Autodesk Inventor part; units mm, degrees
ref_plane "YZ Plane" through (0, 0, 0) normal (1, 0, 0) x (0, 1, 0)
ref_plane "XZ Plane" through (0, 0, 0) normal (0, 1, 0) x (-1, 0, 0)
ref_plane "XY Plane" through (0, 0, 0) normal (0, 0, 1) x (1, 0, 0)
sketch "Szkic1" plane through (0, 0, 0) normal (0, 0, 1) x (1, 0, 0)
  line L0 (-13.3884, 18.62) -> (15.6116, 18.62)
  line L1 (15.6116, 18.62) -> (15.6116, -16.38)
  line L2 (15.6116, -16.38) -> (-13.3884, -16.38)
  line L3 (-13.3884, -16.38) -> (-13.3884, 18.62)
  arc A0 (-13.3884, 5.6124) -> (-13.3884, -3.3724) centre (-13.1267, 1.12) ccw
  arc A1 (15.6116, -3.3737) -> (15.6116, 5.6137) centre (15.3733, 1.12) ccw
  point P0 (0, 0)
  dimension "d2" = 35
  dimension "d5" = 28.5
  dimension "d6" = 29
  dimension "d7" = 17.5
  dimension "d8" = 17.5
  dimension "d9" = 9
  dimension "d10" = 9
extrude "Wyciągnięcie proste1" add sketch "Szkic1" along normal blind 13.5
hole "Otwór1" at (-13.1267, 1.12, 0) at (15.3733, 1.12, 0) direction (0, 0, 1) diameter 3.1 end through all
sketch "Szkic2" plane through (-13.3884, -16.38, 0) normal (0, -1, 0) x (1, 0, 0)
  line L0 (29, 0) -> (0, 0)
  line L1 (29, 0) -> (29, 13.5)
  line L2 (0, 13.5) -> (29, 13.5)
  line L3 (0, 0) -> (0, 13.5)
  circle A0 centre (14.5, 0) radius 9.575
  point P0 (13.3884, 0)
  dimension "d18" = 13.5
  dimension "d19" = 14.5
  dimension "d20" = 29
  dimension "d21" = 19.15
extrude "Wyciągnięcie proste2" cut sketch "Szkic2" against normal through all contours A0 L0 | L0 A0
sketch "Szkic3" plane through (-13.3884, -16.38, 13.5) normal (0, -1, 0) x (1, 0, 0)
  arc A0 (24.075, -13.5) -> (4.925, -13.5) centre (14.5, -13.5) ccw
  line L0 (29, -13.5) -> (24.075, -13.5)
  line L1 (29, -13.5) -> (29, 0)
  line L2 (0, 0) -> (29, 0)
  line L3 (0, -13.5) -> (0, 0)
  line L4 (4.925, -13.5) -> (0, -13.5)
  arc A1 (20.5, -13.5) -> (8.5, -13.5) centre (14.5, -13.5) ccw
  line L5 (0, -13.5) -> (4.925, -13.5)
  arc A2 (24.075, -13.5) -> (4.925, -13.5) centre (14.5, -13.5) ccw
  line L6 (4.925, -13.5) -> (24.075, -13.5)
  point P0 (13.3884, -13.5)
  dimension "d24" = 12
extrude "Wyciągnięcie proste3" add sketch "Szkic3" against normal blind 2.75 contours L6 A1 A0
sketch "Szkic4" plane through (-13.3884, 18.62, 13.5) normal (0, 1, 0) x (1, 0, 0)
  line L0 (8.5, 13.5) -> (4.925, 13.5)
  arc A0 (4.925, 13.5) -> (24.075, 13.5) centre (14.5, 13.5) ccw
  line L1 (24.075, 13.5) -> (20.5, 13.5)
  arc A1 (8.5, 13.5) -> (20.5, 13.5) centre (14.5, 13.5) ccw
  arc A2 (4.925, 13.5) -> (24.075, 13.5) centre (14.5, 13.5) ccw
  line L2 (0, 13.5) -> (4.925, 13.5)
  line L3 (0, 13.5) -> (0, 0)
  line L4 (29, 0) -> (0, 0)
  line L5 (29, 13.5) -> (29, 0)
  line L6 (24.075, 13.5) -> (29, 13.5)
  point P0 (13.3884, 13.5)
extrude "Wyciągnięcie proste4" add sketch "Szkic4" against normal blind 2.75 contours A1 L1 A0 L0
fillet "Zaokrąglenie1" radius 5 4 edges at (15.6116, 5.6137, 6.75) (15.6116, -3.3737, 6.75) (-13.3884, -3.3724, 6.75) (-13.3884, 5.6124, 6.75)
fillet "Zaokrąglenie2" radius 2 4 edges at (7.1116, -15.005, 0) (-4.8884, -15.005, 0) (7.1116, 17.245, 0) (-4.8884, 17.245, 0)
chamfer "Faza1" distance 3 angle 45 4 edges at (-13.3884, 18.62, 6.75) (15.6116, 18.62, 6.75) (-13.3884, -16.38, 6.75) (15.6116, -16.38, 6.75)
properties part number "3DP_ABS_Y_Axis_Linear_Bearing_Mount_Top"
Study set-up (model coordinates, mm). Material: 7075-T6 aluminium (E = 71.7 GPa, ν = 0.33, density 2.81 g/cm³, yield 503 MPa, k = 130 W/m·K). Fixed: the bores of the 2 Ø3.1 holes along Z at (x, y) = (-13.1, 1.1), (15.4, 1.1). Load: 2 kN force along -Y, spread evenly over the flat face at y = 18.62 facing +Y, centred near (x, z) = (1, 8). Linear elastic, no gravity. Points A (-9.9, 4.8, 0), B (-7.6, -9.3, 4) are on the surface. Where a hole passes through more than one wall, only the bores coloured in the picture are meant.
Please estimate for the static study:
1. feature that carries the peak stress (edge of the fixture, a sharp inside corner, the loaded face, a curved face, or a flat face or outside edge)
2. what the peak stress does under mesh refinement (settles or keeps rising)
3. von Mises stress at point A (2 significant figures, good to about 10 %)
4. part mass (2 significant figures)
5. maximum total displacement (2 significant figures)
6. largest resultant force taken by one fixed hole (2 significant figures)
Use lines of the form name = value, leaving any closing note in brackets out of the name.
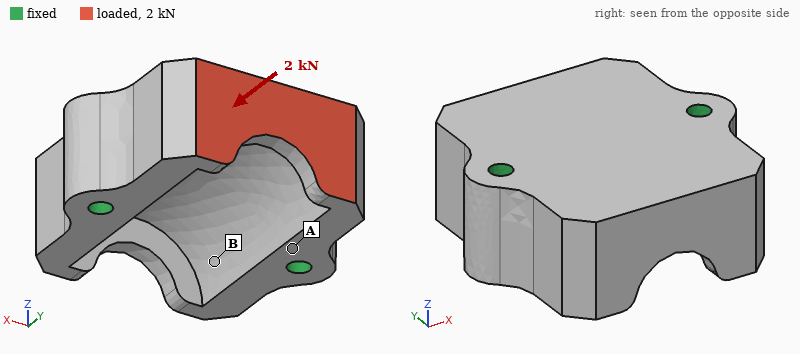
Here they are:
feature that carries the peak stress = a sharp inside corner
what the peak stress does under mesh refinement = keeps rising
von Mises stress at point A = 8.1 MPa
part mass = 27 g
maximum total displacement = 8.6 µm
largest resultant force taken by one fixed hole = 1.0 kN
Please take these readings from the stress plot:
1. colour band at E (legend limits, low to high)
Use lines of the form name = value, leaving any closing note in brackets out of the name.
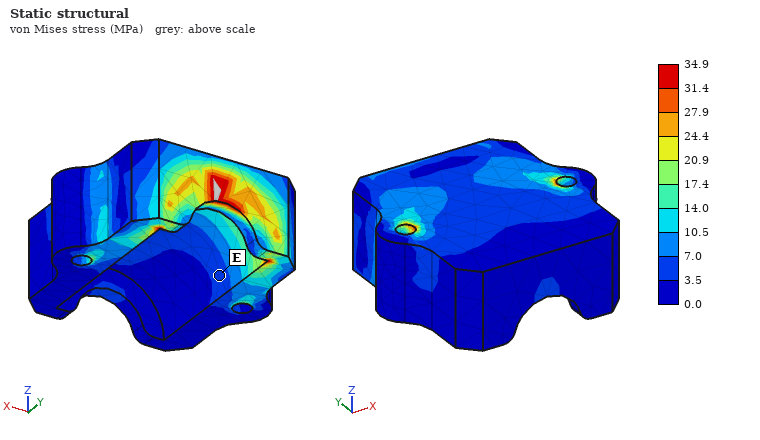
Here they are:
colour band at E = 3.5 to 7.0 MPa
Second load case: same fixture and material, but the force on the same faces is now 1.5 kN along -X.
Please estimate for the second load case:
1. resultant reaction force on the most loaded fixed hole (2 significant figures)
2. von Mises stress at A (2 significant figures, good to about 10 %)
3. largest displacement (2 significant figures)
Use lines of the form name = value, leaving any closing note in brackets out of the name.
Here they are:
resultant reaction force on the most loaded fixed hole = 1.1 kN
von Mises stress at A = 14 MPa
largest displacement = 15 µm
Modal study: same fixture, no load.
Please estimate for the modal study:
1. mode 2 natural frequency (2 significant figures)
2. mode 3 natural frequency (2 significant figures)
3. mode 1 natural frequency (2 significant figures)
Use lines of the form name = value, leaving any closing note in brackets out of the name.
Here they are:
mode 2 natural frequency = 24 kHz
mode 3 natural frequency = 25 kHz
mode 1 natural frequency = 20 kHz
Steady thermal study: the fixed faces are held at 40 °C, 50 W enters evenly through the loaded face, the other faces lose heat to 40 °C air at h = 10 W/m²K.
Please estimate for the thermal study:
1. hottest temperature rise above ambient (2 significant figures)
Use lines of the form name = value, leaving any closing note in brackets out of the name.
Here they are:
hottest temperature rise above ambient = 35 K
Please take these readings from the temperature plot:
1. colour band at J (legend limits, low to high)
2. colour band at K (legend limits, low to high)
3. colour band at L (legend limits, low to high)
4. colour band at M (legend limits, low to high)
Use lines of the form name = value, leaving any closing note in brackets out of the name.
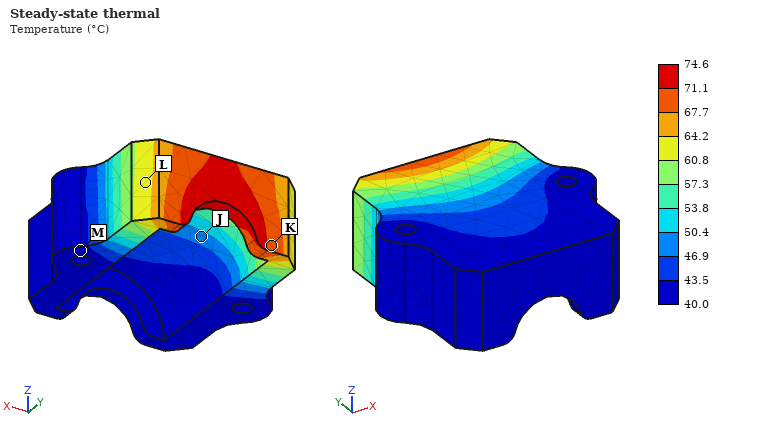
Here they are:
colour band at J = 46.9 to 50.4 °C
colour band at K = 67.7 to 71.1 °C
colour band at L = 60.8 to 64.2 °C
colour band at M = 40.0 to 43.5 °C
